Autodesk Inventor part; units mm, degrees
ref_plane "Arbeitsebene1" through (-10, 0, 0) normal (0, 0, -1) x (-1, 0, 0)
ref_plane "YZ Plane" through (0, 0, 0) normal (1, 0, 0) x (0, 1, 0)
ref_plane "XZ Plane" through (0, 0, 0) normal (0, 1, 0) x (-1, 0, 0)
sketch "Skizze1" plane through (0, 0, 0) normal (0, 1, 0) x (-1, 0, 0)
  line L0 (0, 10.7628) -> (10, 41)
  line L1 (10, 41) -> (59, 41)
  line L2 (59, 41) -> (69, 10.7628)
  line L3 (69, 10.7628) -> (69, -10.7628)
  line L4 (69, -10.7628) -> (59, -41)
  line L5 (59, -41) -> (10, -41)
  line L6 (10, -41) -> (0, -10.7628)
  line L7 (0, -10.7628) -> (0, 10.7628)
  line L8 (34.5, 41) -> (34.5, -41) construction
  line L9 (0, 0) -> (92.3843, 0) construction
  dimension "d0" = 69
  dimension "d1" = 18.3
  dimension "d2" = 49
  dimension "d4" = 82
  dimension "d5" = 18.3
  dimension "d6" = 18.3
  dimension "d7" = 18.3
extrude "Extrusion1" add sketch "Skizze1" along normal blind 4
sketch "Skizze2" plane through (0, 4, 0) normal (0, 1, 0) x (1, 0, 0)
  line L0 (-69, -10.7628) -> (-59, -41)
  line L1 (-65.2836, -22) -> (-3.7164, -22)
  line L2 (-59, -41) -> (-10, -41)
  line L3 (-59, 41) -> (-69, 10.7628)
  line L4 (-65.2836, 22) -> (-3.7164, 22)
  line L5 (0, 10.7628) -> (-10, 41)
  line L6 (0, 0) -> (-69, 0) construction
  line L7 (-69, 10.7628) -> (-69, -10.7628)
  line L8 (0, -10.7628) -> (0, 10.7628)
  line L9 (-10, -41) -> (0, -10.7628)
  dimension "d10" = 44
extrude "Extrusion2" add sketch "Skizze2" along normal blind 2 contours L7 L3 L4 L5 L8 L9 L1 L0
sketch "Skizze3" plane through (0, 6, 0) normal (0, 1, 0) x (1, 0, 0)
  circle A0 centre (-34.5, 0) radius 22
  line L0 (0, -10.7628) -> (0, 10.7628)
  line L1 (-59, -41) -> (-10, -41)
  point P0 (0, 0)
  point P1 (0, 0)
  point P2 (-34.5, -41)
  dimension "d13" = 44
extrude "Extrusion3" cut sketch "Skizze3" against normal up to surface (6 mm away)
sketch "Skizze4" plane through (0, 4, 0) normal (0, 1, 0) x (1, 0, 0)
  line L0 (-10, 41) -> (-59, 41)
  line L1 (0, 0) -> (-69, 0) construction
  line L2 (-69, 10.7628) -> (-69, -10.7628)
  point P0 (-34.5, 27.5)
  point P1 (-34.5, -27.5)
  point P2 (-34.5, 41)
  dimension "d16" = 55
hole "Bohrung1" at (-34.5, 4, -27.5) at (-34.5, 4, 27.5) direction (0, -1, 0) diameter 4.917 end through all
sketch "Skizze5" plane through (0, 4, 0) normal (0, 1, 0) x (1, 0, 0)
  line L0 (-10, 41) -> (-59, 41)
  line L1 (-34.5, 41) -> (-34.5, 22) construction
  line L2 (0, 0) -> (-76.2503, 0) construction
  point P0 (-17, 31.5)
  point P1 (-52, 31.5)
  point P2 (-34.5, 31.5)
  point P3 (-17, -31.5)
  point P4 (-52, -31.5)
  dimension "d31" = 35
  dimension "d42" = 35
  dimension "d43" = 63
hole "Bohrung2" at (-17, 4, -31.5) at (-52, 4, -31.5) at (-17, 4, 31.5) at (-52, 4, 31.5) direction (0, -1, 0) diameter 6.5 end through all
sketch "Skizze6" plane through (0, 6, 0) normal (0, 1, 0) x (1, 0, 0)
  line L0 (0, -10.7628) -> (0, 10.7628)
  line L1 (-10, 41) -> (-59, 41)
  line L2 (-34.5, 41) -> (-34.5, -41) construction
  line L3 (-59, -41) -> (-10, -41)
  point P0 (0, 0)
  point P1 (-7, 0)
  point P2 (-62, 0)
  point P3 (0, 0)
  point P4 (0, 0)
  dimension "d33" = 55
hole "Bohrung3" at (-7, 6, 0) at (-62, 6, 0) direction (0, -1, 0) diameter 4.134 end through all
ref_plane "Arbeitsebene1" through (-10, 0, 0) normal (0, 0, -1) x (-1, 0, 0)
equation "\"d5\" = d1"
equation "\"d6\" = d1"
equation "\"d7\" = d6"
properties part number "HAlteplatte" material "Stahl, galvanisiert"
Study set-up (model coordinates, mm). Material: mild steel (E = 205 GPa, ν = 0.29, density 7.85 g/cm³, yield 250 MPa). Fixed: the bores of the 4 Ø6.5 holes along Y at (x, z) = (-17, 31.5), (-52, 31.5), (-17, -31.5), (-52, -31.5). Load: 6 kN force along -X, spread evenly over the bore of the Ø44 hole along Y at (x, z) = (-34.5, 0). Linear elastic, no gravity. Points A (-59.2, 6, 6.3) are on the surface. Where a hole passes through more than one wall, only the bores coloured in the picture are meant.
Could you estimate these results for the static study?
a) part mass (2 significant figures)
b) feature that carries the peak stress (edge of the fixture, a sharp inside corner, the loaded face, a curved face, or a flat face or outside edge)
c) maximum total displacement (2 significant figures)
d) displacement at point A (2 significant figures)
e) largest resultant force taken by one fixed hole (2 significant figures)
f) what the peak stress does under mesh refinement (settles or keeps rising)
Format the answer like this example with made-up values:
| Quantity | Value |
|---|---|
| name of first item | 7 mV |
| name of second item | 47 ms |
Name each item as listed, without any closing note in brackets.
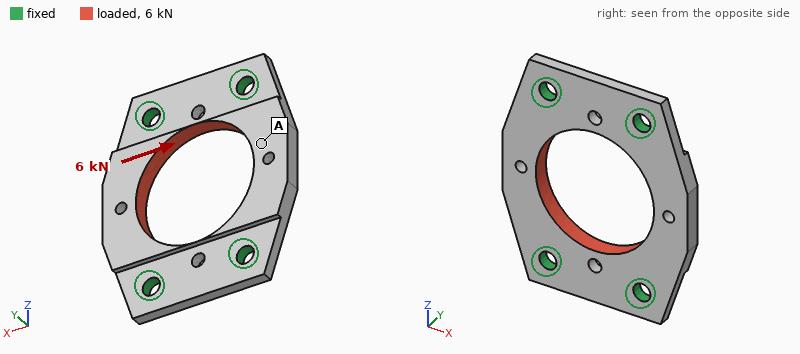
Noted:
| Quantity | Value |
|---|---|
| part mass | 130 g |
| feature that carries the peak stress | a sharp inside corner |
| maximum total displacement | 8.0 µm |
| displacement at point A | 6.9 µm |
| largest resultant force taken by one fixed hole | 1.5 kN |
| what the peak stress does under mesh refinement | keeps rising |
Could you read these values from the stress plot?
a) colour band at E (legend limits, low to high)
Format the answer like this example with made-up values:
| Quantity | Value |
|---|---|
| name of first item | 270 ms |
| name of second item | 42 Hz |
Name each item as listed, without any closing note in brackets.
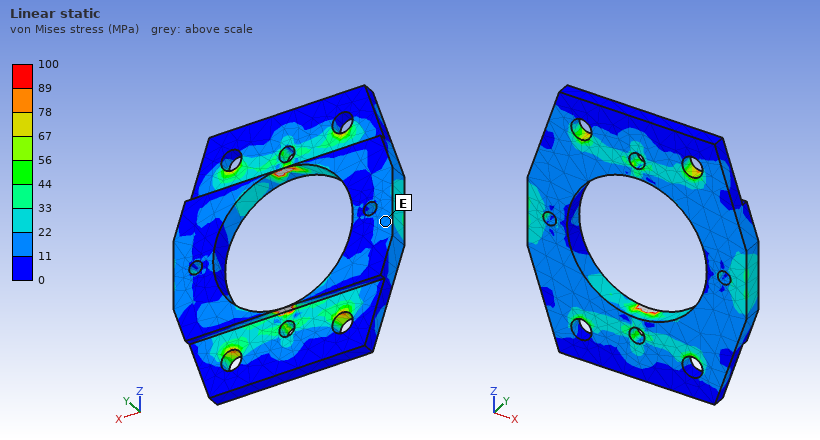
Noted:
| Quantity | Value |
|---|---|
| colour band at E | 11 to 22 MPa |
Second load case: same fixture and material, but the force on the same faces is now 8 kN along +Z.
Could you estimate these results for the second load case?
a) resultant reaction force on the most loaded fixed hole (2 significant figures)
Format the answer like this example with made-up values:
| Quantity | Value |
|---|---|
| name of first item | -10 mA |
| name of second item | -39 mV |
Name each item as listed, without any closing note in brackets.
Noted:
| Quantity | Value |
|---|---|
| resultant reaction force on the most loaded fixed hole | 2.0 kN |
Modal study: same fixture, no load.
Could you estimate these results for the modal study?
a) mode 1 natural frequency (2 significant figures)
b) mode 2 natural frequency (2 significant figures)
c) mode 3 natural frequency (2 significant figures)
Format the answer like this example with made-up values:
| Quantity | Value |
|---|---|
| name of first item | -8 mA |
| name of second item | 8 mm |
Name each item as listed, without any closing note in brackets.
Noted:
| Quantity | Value |
|---|---|
| mode 1 natural frequency | 5500 Hz |
| mode 2 natural frequency | 5600 Hz |
| mode 3 natural frequency | 15 kHz |
